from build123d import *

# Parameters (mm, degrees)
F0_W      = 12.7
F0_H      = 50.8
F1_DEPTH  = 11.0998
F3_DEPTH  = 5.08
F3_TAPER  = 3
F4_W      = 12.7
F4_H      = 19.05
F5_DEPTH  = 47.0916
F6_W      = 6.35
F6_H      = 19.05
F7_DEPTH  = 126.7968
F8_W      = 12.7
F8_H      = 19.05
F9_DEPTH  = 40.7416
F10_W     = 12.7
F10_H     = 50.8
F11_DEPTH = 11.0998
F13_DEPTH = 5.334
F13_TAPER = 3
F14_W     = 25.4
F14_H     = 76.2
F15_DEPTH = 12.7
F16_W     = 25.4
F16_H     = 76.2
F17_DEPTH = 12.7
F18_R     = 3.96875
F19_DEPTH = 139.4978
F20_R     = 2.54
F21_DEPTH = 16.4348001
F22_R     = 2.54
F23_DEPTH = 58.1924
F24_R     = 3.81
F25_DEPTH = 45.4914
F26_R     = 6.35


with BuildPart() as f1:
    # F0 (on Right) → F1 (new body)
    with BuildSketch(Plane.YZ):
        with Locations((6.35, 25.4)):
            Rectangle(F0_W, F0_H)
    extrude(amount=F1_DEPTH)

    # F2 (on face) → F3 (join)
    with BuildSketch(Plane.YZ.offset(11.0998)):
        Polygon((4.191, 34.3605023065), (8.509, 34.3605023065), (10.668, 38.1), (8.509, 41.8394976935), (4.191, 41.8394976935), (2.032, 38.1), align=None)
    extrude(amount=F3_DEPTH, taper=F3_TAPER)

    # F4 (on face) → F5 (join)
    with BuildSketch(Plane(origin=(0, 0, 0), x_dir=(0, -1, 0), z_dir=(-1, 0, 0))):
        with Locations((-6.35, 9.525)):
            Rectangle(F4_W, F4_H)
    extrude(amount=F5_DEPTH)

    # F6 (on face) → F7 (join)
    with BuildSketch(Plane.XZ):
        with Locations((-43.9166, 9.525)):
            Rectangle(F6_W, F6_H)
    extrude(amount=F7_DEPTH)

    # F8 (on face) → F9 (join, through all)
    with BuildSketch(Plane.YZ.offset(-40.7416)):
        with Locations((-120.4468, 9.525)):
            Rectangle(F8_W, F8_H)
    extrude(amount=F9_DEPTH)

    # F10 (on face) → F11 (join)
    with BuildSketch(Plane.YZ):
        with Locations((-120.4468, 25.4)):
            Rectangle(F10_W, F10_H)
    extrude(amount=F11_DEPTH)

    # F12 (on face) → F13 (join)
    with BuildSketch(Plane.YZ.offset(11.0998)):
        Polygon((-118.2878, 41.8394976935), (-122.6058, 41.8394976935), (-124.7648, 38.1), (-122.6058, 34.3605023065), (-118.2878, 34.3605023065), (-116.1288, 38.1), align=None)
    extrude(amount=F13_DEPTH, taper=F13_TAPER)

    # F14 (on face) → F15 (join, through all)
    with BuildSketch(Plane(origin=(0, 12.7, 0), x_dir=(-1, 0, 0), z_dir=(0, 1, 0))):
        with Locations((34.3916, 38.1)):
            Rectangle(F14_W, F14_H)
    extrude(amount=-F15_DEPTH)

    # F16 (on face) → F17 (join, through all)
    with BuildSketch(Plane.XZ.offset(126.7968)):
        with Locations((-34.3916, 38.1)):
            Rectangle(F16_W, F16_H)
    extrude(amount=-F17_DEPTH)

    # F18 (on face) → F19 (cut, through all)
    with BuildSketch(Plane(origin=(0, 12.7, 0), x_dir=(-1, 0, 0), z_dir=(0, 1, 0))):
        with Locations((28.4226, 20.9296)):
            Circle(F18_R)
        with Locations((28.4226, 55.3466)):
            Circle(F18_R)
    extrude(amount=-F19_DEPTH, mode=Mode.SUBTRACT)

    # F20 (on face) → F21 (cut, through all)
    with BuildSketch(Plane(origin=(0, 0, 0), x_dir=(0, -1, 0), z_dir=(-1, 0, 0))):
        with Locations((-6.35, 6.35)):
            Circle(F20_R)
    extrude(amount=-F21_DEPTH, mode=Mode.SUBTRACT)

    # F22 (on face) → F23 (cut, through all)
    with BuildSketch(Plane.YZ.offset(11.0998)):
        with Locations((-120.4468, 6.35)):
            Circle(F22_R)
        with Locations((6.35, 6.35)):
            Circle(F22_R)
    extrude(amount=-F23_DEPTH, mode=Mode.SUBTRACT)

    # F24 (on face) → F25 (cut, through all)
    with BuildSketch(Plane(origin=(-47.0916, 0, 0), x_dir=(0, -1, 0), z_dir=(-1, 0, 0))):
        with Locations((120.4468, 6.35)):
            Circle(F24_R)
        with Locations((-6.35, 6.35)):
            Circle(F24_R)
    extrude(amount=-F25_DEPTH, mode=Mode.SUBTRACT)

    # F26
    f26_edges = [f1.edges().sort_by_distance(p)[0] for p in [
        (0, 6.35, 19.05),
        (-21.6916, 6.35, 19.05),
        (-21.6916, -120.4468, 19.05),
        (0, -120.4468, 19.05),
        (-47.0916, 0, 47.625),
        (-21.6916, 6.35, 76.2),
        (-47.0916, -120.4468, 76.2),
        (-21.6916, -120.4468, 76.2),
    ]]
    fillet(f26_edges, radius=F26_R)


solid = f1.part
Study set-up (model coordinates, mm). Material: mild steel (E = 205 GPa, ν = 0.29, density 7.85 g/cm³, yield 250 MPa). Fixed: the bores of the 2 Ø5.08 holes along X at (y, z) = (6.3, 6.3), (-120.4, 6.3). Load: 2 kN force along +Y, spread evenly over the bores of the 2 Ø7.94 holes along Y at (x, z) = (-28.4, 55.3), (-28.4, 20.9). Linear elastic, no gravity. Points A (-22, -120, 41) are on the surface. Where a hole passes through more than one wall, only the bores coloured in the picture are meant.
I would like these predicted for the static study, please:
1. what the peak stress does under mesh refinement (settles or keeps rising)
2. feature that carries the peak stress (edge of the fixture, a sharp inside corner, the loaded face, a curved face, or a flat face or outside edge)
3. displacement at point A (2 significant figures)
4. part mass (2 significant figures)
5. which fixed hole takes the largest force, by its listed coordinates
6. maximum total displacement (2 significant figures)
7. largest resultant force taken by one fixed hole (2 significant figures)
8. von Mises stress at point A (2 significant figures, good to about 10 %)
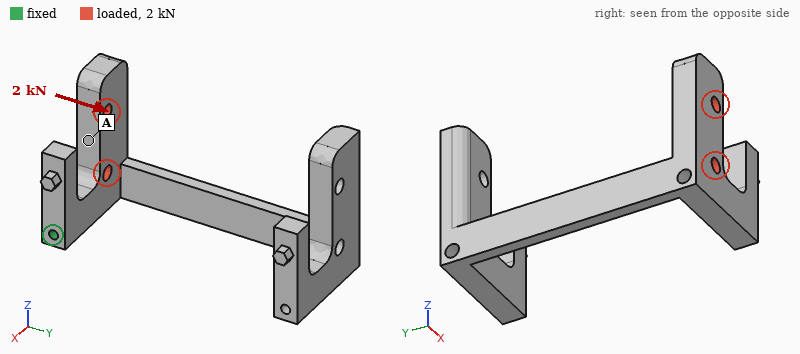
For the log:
keeps rising
edge of the fixture
0.11 mm
630 g
(-120.4, 6.3)
0.23 mm
1.7 kN
20 MPa
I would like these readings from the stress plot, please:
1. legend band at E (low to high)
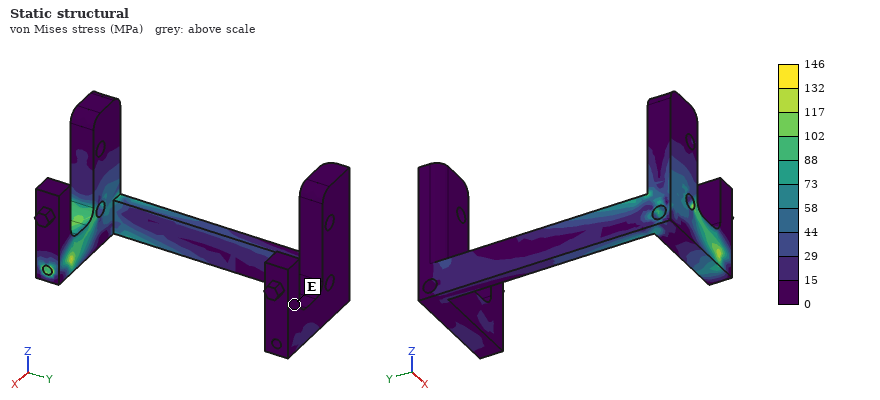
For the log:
0 to 15 MPa
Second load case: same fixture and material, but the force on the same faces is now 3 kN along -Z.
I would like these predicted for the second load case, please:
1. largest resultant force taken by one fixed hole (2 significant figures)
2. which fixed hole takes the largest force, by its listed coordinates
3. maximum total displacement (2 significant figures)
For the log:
2.9 kN
(-120.4, 6.3)
0.13 mm
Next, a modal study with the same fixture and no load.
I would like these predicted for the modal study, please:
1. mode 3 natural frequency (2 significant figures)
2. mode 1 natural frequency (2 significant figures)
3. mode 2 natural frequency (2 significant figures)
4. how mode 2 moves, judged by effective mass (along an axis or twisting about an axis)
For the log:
1300 Hz
680 Hz
1100 Hz
along Y
